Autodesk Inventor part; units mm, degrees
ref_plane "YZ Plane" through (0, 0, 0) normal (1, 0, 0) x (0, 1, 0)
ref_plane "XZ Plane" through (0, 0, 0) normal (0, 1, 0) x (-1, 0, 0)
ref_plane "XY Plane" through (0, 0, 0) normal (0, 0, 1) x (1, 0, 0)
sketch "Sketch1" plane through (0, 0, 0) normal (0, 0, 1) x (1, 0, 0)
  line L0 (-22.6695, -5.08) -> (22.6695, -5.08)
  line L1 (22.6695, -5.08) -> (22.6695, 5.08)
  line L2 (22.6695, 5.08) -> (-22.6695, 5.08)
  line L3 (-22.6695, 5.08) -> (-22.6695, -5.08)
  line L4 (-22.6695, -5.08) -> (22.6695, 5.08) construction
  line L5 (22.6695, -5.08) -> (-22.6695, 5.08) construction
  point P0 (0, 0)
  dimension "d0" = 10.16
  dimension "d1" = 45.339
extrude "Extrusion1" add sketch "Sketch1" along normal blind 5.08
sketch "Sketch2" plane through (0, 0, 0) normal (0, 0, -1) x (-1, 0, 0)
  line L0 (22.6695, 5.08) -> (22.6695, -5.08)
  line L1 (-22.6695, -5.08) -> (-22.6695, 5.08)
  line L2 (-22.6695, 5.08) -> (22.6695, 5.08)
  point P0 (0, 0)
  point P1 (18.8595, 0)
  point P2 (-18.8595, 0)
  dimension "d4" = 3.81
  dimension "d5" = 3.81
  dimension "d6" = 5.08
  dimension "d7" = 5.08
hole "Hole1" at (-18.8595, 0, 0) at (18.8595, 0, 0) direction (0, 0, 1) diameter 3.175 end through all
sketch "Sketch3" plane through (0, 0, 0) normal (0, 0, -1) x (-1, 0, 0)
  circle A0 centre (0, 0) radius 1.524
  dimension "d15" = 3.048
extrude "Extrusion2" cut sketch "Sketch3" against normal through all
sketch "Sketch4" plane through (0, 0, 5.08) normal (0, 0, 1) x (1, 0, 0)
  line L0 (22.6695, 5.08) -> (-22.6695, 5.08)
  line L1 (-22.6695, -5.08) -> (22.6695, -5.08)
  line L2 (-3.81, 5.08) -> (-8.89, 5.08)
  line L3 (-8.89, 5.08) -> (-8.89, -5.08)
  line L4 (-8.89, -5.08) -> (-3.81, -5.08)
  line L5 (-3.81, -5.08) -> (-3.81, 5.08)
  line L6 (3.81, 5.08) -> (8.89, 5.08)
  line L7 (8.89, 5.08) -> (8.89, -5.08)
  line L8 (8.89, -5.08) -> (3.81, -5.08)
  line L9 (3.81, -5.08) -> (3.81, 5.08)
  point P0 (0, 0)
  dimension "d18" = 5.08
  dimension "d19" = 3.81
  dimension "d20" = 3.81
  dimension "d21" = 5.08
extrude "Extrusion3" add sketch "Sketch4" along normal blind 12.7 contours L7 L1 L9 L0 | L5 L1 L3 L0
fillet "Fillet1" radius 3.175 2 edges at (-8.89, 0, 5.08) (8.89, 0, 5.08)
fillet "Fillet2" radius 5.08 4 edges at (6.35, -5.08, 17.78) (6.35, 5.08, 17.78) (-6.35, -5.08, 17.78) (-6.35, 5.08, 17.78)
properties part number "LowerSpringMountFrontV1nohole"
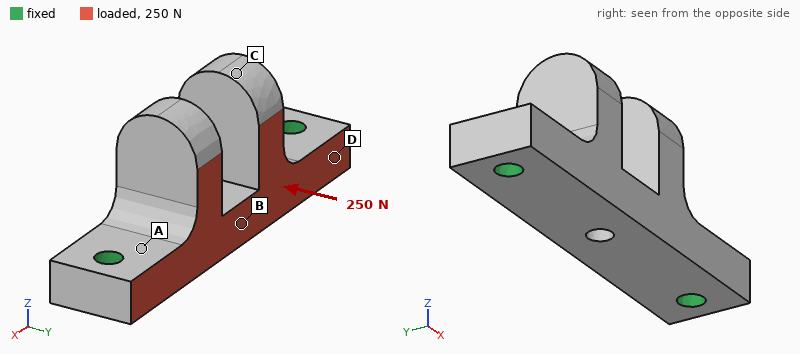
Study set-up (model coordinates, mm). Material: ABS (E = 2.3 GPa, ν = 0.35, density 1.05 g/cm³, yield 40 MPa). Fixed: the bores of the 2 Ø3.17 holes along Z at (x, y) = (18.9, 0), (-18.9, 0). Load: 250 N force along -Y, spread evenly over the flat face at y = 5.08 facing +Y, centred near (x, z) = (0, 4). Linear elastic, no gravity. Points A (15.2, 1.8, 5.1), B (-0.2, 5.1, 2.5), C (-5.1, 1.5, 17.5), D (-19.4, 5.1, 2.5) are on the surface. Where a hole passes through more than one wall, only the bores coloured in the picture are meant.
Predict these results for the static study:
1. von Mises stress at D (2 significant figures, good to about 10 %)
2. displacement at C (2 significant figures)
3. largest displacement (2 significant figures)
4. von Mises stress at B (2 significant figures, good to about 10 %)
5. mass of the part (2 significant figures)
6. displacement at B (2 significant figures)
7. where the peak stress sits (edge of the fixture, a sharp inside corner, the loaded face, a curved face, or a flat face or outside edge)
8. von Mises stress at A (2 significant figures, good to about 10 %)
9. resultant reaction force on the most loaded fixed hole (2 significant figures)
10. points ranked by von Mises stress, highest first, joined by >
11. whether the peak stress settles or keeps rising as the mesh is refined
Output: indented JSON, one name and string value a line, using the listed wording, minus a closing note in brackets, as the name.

{
  "von Mises stress at D": "3.4 MPa",
  "displacement at C": "0.19 mm",
  "largest displacement": "0.19 mm",
  "von Mises stress at B": "6.3 MPa",
  "mass of the part": "3.6 g",
  "displacement at B": "0.089 mm",
  "where the peak stress sits": "edge of the fixture",
  "von Mises stress at A": "8.5 MPa",
  "resultant reaction force on the most loaded fixed hole": "130 N",
  "points ranked by von Mises stress, highest first, joined by >": "A > B > D > C",
  "whether the peak stress settles or keeps rising as the mesh is refined": "keeps rising"
}
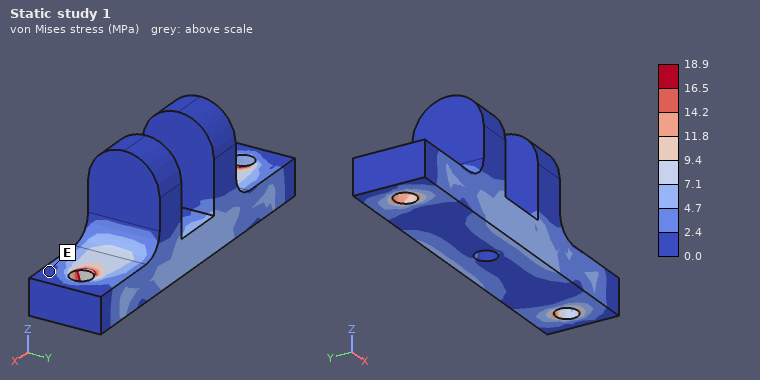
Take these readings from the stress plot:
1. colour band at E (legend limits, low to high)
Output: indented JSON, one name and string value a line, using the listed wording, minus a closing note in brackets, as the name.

{
  "colour band at E": "0.0 to 2.4 MPa"
}
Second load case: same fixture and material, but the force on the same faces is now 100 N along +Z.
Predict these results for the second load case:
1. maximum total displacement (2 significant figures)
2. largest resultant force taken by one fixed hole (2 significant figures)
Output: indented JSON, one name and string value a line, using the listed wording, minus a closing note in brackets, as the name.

{
  "maximum total displacement": "0.13 mm",
  "largest resultant force taken by one fixed hole": "50 N"
}
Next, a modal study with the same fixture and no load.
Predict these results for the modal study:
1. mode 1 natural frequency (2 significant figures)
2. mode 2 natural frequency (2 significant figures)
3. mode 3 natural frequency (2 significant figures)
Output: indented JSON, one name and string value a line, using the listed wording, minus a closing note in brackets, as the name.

{
  "mode 1 natural frequency": "3000 Hz",
  "mode 2 natural frequency": "3100 Hz",
  "mode 3 natural frequency": "5000 Hz"
}
